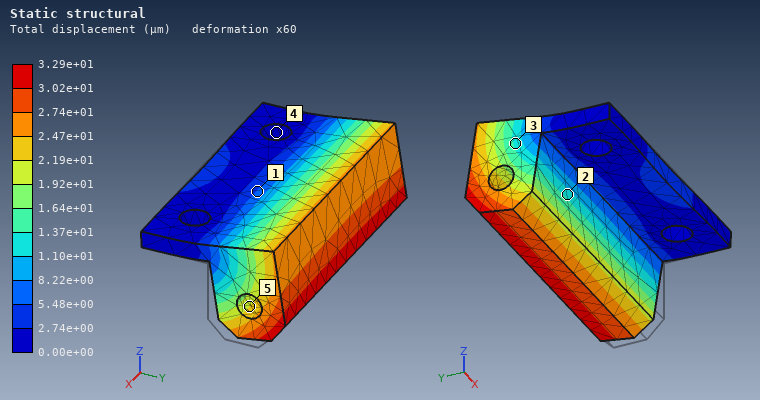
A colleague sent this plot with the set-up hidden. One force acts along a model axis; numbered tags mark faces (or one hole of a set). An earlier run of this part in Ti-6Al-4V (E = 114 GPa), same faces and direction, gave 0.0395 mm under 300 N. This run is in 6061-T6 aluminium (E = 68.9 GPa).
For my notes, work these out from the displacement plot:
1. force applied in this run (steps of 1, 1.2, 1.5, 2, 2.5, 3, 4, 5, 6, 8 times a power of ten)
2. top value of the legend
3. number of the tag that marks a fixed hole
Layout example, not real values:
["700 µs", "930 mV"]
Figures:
["150 N", "3.29e+01 µm", "4"]
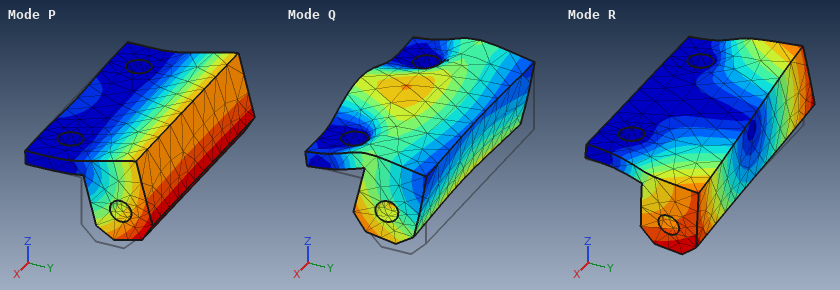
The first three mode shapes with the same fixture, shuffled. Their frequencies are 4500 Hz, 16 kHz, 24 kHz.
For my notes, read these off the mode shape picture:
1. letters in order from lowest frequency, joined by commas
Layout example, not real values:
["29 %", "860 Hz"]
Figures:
["P, R, Q"]
